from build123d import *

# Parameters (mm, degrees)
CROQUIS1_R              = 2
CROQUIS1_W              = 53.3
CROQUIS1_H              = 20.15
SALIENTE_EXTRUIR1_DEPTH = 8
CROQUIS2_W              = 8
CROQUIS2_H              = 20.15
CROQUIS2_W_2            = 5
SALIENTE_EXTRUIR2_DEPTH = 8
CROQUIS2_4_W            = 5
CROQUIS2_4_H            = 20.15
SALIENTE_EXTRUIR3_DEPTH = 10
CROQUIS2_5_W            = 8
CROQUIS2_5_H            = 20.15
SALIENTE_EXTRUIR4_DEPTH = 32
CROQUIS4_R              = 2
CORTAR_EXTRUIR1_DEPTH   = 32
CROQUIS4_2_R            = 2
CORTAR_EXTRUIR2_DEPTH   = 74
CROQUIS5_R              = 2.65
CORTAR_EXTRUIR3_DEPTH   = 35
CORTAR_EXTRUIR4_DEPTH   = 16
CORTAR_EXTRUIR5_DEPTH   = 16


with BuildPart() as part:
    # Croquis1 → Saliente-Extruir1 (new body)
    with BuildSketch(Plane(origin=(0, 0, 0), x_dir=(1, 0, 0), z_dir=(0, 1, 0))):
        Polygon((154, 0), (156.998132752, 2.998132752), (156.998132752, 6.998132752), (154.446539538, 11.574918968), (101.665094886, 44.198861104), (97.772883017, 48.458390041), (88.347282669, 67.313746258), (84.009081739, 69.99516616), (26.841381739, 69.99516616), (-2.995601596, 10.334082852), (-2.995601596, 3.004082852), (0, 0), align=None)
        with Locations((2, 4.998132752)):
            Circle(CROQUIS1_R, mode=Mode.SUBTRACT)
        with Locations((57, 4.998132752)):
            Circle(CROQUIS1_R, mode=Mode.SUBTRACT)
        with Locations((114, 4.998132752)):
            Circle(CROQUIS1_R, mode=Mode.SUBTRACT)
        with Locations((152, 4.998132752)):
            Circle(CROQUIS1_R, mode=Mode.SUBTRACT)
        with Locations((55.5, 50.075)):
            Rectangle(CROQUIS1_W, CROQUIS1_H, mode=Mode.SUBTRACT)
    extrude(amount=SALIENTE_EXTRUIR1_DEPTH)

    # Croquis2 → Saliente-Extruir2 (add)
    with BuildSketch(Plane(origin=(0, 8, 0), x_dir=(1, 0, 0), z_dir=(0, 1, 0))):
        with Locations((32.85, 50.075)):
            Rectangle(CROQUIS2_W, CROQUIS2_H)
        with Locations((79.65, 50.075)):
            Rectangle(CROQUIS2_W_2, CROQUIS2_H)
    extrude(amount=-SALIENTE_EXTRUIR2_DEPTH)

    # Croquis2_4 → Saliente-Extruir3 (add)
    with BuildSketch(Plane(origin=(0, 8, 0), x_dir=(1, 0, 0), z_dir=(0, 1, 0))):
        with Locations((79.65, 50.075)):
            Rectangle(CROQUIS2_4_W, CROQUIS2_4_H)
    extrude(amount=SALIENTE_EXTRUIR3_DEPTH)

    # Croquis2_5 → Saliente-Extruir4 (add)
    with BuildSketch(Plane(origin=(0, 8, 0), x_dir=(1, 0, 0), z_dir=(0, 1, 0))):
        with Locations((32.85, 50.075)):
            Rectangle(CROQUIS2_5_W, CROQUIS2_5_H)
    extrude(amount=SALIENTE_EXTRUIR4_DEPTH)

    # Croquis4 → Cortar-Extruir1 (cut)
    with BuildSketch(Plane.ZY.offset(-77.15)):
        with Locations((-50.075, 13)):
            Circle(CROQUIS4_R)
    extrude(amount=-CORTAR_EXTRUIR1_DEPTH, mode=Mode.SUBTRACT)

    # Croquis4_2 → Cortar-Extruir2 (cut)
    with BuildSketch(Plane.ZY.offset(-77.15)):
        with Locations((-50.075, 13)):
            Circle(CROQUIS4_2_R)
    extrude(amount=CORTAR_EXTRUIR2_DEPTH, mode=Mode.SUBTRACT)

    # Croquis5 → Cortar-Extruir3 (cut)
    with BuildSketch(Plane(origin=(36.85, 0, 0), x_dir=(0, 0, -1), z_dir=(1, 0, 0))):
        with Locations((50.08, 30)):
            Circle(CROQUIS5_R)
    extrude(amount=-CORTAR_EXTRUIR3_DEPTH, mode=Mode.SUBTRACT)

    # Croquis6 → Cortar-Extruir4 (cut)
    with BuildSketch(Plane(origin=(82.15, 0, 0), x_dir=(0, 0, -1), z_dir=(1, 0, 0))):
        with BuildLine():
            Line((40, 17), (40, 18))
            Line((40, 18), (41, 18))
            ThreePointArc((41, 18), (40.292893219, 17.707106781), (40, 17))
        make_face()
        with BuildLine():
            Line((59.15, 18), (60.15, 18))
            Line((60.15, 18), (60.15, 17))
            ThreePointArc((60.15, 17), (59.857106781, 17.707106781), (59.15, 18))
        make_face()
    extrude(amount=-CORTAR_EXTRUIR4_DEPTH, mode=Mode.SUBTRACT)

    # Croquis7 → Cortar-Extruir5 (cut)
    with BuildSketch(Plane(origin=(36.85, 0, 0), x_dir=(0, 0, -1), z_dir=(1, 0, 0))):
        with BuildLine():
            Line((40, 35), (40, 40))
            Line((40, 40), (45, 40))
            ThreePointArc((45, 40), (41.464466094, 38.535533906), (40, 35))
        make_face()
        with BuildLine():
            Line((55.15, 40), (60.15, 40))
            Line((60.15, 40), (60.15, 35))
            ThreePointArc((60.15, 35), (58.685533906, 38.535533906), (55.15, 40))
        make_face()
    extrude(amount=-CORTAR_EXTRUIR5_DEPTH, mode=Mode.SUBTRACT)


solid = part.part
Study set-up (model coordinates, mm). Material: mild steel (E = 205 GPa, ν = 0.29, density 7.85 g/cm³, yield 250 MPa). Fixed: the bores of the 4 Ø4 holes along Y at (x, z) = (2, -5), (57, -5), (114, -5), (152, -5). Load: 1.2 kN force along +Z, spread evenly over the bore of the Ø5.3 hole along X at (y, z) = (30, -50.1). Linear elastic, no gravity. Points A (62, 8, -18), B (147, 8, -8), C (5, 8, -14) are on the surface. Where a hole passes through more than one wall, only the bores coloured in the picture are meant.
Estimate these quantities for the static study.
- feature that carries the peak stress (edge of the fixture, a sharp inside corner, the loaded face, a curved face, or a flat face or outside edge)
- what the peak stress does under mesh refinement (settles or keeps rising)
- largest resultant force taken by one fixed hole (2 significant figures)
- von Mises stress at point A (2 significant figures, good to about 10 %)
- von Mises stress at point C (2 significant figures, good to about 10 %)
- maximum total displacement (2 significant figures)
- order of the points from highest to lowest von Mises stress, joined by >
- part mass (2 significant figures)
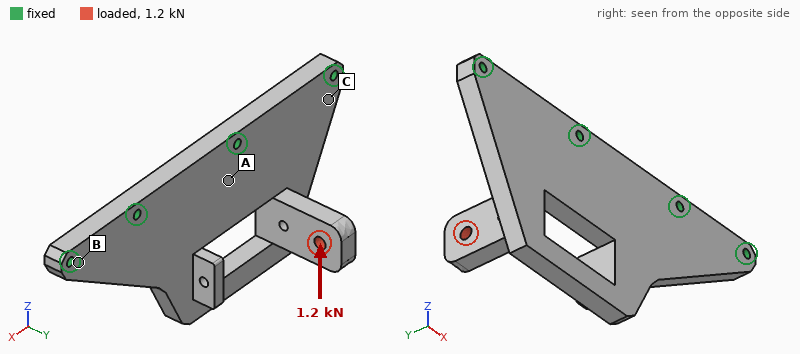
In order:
edge of the fixture
keeps rising
670 N
24 MPa
54 MPa
0.16 mm
C > A > B
480 g
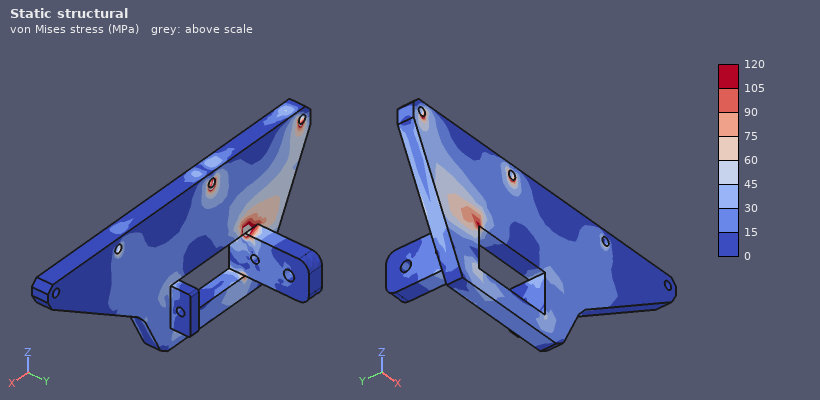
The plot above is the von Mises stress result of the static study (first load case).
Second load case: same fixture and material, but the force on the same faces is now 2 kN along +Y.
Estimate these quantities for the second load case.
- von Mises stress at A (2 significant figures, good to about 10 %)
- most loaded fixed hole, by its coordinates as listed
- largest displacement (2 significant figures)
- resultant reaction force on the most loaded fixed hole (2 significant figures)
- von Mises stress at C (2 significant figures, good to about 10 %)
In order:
59 MPa
(57, -5)
0.25 mm
1.3 kN
120 MPa
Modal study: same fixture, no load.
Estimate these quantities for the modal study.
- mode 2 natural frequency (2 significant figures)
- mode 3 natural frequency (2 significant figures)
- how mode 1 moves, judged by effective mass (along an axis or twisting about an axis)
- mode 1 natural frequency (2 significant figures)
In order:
2800 Hz
4000 Hz
along Y
1400 Hz
